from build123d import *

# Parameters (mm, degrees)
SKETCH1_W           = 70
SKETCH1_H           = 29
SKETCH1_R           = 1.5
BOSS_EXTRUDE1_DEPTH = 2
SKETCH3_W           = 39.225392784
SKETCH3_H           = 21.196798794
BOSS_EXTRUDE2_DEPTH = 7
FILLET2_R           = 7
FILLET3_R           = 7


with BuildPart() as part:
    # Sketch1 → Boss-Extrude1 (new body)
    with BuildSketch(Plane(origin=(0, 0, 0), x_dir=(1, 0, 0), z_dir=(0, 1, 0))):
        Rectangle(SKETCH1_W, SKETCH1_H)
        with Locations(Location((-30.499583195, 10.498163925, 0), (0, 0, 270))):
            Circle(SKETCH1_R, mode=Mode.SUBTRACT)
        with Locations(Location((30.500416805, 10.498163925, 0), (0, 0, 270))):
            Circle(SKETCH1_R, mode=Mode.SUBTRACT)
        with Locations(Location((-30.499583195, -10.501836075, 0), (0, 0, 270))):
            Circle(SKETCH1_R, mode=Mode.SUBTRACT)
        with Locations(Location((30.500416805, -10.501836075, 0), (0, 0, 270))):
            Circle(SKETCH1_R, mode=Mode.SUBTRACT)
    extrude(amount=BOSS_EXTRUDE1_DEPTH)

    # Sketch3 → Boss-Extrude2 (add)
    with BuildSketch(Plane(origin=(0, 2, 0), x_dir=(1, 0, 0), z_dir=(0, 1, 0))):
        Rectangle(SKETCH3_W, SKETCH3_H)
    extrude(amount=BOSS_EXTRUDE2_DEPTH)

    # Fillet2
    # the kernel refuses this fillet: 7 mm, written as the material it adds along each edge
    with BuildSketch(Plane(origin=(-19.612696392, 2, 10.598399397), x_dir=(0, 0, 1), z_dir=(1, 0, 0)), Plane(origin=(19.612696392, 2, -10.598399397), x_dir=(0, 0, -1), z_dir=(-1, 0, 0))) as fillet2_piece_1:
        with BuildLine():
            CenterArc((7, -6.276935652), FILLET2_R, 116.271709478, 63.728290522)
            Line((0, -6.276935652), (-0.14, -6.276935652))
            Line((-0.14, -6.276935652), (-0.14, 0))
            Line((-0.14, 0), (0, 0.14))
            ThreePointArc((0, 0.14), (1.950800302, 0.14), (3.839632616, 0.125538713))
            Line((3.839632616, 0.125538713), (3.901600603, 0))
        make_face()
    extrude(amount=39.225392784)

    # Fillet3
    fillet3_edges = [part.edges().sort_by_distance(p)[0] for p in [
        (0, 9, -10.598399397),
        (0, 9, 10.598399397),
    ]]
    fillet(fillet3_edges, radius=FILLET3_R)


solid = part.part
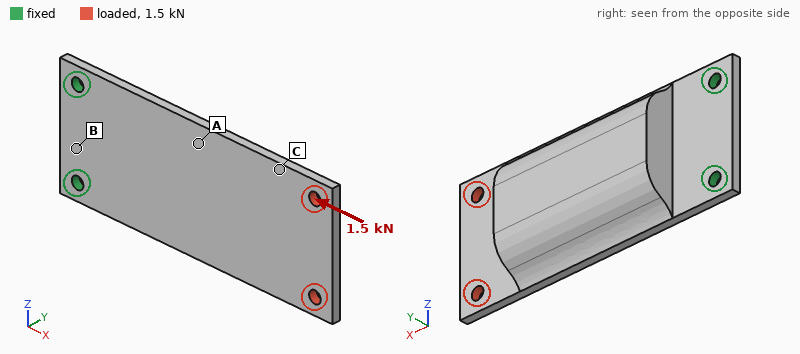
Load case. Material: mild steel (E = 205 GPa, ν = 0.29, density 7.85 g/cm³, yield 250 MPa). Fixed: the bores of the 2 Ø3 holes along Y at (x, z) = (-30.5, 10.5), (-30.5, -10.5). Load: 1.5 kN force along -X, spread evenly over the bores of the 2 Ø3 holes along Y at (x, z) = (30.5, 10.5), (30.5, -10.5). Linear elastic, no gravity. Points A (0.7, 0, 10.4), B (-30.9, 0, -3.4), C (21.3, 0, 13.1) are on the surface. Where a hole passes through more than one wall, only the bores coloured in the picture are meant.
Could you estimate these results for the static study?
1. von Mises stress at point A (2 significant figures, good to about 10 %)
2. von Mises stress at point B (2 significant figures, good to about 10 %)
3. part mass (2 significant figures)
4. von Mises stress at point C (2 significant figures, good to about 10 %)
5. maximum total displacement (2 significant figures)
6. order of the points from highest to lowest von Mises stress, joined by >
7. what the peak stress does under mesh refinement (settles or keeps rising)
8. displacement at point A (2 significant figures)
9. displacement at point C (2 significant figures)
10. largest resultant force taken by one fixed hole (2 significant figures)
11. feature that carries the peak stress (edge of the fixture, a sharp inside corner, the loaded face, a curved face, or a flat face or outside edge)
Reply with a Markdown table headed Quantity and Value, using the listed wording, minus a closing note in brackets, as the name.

| Quantity | Value |
|---|---|
| von Mises stress at point A | 21 MPa |
| von Mises stress at point B | 9.4 MPa |
| part mass | 78 g |
| von Mises stress at point C | 34 MPa |
| maximum total displacement | 30 µm |
| order of the points from highest to lowest von Mises stress, joined by > | C > A > B |
| what the peak stress does under mesh refinement | keeps rising |
| displacement at point A | 6.4 µm |
| displacement at point C | 19 µm |
| largest resultant force taken by one fixed hole | 760 N |
| feature that carries the peak stress | edge of the fixture |
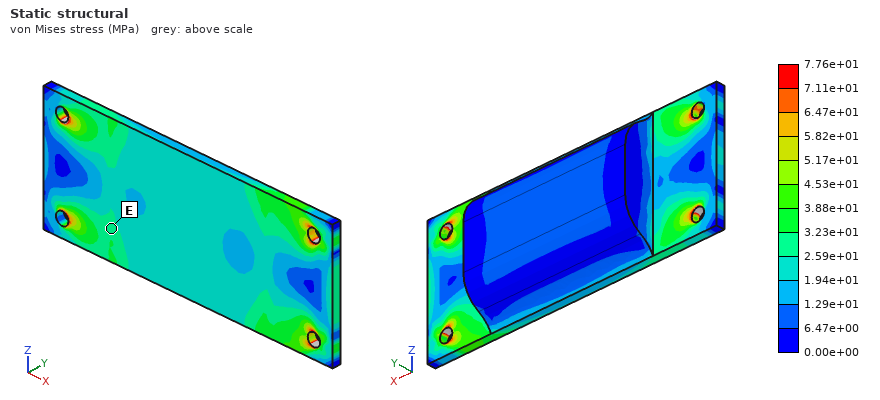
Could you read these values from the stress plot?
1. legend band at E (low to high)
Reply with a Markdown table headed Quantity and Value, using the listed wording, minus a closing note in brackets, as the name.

| Quantity | Value |
|---|---|
| legend band at E | 2.59e+01 to 3.23e+01 MPa |
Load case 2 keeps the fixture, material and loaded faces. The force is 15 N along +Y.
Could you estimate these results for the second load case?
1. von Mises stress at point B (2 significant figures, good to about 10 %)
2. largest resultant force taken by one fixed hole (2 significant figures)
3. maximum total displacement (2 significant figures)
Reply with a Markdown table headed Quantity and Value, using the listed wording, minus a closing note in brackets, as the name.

| Quantity | Value |
|---|---|
| von Mises stress at point B | 16 MPa |
| largest resultant force taken by one fixed hole | 8.2 N |
| maximum total displacement | 0.15 mm |
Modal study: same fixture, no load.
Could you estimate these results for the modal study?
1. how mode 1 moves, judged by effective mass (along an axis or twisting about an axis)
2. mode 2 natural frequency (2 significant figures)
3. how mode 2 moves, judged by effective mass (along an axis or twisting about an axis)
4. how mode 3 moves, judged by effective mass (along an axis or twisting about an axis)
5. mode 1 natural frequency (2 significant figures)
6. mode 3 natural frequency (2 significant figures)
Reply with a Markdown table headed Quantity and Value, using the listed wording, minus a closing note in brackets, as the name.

| Quantity | Value |
|---|---|
| how mode 1 moves, judged by effective mass | along Y |
| mode 2 natural frequency | 3400 Hz |
| how mode 2 moves, judged by effective mass | along Z |
| how mode 3 moves, judged by effective mass | along Z |
| mode 1 natural frequency | 360 Hz |
| mode 3 natural frequency | 4000 Hz |
